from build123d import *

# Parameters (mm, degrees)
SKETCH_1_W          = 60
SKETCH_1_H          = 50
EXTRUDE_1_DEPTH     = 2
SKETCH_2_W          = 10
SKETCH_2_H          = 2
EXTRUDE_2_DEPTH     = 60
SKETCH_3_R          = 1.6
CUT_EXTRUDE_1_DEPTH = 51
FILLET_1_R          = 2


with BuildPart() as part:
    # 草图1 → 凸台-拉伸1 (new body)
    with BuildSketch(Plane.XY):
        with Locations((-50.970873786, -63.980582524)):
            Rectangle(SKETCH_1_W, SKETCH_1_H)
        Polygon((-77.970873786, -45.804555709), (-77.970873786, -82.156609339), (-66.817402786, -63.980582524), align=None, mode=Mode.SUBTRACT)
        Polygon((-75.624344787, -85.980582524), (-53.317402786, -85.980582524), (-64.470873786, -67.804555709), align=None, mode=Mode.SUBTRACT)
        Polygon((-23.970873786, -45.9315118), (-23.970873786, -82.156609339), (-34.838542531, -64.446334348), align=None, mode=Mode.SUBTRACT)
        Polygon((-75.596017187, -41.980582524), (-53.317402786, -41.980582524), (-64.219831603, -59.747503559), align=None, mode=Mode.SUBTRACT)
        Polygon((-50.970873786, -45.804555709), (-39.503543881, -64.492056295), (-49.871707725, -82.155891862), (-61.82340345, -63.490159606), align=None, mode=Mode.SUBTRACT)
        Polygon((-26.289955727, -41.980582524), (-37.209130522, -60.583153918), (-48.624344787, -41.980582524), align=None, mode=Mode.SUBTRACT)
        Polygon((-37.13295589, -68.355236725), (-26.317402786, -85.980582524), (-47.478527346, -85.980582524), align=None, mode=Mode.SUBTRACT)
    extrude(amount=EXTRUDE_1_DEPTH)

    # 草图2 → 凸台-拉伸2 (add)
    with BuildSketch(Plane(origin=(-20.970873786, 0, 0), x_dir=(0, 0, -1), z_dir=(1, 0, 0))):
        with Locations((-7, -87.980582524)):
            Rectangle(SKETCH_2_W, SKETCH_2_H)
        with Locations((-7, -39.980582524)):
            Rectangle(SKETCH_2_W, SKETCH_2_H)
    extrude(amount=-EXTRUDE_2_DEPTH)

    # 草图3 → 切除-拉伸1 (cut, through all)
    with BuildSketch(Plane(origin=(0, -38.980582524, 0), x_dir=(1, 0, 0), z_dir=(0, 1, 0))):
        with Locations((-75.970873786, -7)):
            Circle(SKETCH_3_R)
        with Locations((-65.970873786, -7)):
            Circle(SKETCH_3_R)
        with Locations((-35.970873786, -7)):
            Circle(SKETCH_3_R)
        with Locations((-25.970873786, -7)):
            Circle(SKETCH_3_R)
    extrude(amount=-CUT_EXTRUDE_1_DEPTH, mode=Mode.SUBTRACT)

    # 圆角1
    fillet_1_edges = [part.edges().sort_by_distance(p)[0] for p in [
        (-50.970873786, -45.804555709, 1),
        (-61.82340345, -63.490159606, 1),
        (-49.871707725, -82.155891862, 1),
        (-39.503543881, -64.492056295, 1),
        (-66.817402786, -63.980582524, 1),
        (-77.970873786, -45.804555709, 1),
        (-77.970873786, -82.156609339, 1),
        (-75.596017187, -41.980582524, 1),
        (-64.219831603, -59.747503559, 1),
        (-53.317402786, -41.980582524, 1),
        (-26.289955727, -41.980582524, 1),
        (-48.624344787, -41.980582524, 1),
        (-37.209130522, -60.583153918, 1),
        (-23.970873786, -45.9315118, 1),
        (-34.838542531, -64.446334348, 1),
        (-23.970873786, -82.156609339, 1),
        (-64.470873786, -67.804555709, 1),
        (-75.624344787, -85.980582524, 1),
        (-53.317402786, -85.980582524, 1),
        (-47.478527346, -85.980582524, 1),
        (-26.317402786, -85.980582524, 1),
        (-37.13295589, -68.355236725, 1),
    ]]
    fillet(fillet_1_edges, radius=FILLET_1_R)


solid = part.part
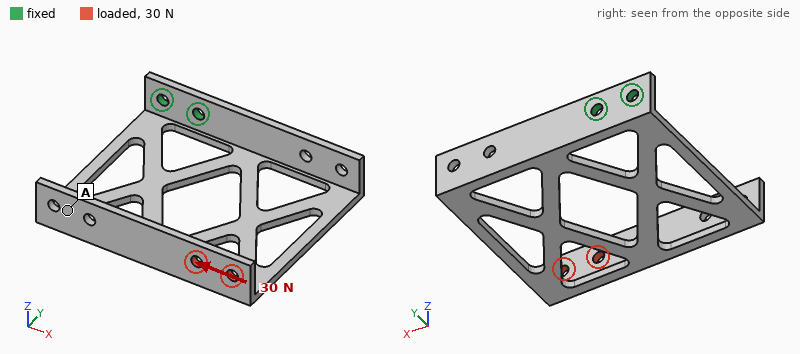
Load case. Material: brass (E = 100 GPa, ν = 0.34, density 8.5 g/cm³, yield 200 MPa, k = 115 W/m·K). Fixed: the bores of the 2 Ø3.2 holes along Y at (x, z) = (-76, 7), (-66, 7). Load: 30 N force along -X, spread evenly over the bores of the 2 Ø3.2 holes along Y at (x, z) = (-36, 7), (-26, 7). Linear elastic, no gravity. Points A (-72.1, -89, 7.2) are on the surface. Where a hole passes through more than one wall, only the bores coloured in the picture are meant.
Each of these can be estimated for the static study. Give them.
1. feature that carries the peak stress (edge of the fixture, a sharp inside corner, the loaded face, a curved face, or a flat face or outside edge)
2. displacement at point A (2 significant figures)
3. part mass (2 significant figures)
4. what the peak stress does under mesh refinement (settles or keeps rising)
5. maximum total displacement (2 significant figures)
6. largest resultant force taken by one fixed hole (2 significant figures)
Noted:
edge of the fixture
0.10 mm
44 g
keeps rising
0.21 mm
93 N
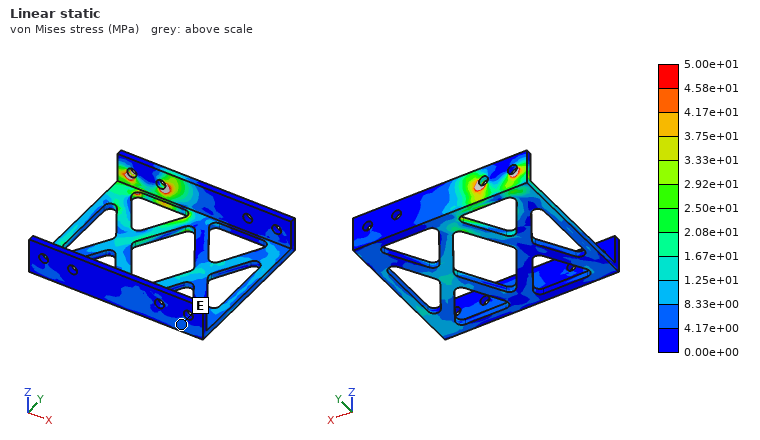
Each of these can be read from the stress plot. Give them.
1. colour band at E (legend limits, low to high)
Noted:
4.17e+00 to 8.33e+00 MPa
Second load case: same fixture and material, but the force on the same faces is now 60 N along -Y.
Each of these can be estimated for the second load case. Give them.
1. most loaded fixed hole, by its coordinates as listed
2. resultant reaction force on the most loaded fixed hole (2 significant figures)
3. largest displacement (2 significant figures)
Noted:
(-66, 7)
170 N
0.48 mm
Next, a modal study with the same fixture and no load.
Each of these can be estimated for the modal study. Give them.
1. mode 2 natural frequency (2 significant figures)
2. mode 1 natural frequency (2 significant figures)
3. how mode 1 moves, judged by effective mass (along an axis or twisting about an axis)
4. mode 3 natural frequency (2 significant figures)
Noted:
470 Hz
190 Hz
along Z
600 Hz
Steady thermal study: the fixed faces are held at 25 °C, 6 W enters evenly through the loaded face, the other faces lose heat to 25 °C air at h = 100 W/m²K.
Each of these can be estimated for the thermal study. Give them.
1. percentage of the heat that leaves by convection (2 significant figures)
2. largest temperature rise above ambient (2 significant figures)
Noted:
92 %
33 K
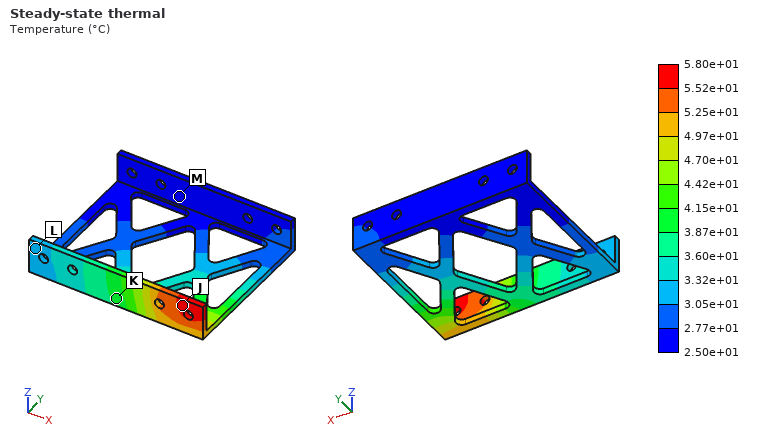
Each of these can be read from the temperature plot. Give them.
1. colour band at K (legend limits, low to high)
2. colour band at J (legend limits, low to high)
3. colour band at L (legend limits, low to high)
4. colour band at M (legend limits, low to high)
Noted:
3.87e+01 to 4.15e+01 °C
5.52e+01 to 5.80e+01 °C
3.05e+01 to 3.32e+01 °C
2.50e+01 to 2.77e+01 °C
